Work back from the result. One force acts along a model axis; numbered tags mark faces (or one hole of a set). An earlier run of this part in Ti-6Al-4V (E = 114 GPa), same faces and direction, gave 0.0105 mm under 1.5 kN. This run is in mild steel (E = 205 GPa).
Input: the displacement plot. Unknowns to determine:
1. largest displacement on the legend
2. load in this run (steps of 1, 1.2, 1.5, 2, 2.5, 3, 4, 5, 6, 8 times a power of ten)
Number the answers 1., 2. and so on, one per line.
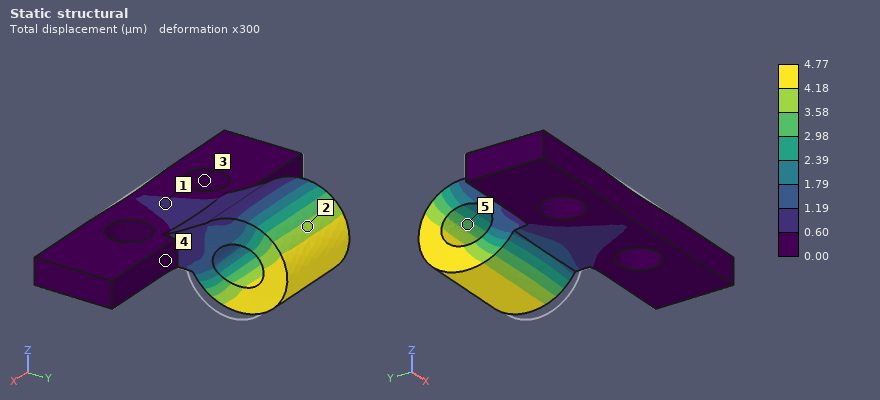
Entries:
1. 4.77 µm
2. 1.2 kN
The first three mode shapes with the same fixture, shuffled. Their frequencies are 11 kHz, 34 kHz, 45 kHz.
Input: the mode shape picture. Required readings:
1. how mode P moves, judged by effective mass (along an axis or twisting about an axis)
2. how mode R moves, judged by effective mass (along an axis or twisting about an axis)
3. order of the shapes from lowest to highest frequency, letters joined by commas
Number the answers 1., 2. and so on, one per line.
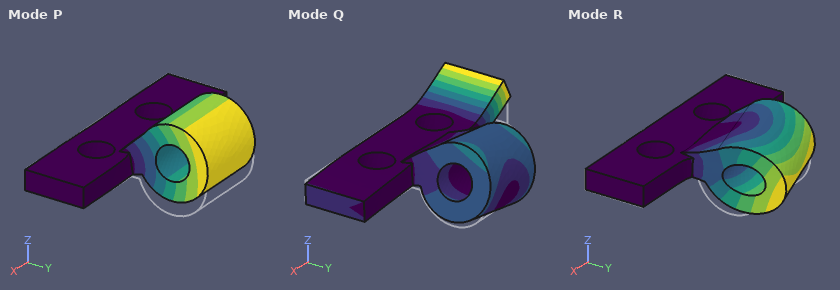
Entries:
1. along Z
2. along X
3. P, R, Q
